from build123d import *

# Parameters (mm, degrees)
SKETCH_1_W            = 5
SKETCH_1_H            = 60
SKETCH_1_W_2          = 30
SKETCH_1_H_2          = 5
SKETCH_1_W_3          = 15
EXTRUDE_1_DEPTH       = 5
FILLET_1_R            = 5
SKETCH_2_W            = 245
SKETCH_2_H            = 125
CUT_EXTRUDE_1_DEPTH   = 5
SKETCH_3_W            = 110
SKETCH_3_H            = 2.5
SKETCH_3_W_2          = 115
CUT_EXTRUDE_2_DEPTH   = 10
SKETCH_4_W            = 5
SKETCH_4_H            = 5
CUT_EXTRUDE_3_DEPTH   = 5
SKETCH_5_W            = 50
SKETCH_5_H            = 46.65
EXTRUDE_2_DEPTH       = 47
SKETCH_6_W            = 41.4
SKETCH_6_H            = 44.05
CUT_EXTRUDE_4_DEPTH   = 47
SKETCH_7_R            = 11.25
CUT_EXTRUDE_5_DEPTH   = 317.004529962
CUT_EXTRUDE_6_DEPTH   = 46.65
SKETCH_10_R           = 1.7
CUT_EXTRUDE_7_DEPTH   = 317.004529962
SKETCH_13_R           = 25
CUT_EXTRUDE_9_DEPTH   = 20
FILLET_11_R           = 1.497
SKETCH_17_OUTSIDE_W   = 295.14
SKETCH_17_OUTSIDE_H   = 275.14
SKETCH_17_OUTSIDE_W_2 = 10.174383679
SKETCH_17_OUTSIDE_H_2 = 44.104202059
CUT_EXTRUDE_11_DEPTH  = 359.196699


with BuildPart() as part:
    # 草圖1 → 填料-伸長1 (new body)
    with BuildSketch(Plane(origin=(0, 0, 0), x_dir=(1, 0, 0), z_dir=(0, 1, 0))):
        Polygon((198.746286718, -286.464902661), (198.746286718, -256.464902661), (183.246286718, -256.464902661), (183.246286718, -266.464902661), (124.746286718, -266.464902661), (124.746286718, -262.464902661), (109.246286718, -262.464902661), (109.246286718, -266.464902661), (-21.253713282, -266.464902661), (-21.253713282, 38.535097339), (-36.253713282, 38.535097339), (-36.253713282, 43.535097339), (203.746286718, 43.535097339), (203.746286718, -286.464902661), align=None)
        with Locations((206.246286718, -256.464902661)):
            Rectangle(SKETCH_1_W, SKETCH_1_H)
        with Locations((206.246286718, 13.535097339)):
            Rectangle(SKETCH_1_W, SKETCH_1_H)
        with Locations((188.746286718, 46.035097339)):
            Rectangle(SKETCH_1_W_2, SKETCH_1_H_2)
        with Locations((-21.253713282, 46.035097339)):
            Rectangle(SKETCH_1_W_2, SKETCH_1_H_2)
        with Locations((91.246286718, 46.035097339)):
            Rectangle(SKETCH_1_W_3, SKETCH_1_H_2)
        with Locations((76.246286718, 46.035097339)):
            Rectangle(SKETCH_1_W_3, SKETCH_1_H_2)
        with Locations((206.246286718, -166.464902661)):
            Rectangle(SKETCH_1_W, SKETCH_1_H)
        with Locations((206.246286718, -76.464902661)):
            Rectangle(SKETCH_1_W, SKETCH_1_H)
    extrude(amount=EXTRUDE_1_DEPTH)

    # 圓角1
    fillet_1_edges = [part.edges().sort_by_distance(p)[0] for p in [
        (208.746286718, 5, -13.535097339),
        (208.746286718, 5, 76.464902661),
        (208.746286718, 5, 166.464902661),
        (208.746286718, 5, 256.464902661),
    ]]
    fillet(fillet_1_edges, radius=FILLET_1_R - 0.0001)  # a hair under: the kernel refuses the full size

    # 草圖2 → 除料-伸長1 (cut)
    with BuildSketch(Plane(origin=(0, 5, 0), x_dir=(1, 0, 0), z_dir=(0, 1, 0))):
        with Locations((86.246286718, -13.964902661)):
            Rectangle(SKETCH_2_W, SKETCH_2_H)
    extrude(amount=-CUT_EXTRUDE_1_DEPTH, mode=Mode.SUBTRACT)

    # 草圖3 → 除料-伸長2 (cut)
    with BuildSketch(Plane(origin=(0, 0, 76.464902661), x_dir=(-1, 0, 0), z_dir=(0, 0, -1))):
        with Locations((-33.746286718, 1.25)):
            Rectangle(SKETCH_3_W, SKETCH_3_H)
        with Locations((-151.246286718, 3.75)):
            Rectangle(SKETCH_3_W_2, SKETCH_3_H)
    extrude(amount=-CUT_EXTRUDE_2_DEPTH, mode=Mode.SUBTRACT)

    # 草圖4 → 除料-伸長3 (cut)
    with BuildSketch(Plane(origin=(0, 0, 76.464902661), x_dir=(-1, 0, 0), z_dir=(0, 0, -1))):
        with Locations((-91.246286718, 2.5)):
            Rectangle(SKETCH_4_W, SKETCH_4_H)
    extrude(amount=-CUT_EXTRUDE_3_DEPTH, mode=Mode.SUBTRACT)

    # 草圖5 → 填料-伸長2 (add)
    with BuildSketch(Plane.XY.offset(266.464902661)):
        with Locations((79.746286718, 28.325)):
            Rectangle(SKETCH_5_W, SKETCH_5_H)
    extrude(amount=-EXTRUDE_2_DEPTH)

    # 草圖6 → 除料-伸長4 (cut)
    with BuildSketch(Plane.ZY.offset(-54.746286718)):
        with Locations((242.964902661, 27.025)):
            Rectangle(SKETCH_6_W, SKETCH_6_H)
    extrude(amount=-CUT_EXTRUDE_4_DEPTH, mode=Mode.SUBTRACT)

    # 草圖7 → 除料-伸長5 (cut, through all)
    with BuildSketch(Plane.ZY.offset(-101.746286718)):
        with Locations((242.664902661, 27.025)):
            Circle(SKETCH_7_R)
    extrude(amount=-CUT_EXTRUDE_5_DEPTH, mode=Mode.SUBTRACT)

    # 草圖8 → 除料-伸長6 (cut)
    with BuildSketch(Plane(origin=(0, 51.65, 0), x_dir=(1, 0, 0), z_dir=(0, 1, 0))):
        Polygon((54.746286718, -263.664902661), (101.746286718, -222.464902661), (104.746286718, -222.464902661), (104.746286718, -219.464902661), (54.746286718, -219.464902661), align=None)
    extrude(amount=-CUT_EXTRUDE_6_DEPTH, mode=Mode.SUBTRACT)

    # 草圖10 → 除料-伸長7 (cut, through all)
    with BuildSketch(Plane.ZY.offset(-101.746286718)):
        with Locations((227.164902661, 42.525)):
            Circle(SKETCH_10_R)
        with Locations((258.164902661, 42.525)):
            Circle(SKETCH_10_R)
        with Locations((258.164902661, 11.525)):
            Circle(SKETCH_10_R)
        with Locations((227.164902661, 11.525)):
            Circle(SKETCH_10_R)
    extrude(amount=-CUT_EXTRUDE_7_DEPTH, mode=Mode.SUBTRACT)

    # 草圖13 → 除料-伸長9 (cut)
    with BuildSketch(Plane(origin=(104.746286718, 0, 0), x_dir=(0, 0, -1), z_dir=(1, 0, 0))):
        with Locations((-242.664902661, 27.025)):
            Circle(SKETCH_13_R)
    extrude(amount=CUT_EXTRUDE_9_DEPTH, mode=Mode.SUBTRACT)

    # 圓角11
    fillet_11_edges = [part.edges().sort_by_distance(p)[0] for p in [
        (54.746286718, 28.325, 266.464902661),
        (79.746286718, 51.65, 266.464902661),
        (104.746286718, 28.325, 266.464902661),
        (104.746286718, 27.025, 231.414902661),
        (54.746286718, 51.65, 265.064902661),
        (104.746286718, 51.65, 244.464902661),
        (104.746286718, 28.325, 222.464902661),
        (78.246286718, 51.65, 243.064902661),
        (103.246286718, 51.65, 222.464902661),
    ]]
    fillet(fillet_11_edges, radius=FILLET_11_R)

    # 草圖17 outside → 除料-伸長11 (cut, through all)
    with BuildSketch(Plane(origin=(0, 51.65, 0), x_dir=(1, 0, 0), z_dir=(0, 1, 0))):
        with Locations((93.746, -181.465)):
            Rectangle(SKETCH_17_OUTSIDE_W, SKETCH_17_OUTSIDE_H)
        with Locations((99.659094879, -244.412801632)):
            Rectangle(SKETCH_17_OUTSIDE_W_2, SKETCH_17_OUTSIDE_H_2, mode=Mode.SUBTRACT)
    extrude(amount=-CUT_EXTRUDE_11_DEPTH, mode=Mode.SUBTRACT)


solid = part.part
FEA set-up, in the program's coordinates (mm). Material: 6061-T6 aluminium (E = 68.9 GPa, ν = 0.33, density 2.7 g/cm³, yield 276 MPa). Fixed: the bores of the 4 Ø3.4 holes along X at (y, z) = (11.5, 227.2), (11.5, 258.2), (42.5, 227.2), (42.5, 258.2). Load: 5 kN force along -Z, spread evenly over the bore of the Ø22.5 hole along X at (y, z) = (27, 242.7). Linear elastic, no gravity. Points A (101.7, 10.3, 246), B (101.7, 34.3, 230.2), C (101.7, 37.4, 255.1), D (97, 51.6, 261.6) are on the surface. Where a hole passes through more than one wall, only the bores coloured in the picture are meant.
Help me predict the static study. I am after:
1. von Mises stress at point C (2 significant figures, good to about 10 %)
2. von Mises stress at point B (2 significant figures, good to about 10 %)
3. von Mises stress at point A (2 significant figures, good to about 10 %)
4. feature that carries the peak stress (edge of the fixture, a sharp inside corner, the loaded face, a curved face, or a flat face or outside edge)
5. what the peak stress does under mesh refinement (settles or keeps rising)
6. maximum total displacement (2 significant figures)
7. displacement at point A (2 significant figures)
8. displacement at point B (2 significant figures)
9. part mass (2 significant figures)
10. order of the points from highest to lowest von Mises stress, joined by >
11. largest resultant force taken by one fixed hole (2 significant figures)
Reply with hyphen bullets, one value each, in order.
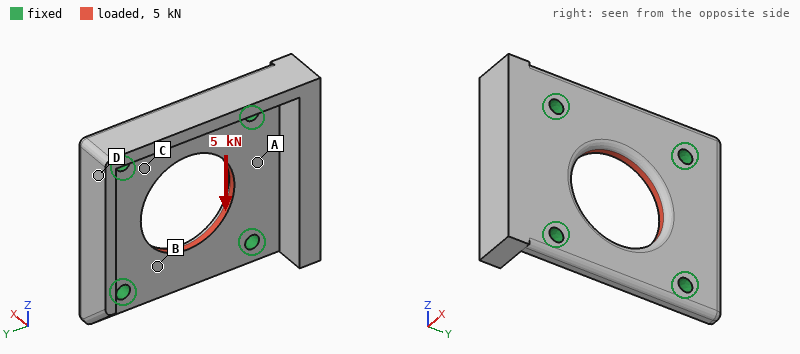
- 45 MPa
- 59 MPa
- 20 MPa
- edge of the fixture
- keeps rising
- 21 µm
- 3.3 µm
- 12 µm
- 23 g
- B > C > A > D
- 1.3 kN
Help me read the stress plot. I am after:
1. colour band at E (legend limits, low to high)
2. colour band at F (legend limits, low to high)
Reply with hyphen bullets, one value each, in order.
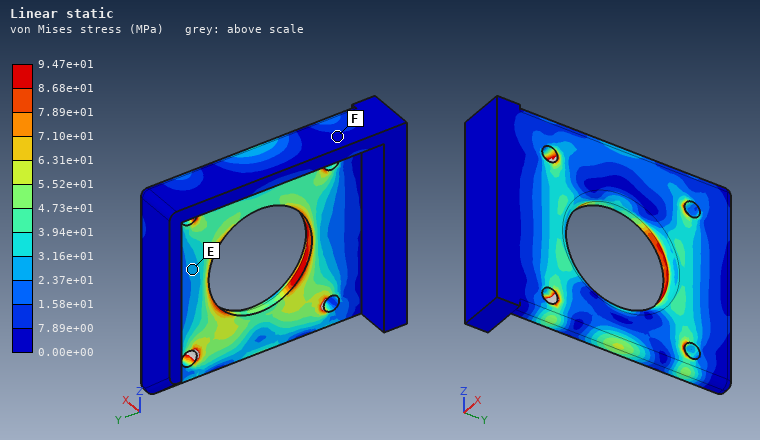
- 2.37e+01 to 3.16e+01 MPa
- 0.00e+00 to 7.89e+00 MPa
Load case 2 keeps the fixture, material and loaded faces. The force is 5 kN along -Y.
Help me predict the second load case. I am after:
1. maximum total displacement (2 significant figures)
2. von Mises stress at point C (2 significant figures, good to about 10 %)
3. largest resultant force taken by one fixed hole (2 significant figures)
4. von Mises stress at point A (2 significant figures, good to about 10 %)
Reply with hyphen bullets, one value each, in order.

- 16 µm
- 42 MPa
- 1.3 kN
- 31 MPa
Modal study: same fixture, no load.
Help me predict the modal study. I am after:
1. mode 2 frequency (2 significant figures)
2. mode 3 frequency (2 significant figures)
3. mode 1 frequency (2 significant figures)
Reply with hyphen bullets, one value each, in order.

- 13 kHz
- 15 kHz
- 8900 Hz
